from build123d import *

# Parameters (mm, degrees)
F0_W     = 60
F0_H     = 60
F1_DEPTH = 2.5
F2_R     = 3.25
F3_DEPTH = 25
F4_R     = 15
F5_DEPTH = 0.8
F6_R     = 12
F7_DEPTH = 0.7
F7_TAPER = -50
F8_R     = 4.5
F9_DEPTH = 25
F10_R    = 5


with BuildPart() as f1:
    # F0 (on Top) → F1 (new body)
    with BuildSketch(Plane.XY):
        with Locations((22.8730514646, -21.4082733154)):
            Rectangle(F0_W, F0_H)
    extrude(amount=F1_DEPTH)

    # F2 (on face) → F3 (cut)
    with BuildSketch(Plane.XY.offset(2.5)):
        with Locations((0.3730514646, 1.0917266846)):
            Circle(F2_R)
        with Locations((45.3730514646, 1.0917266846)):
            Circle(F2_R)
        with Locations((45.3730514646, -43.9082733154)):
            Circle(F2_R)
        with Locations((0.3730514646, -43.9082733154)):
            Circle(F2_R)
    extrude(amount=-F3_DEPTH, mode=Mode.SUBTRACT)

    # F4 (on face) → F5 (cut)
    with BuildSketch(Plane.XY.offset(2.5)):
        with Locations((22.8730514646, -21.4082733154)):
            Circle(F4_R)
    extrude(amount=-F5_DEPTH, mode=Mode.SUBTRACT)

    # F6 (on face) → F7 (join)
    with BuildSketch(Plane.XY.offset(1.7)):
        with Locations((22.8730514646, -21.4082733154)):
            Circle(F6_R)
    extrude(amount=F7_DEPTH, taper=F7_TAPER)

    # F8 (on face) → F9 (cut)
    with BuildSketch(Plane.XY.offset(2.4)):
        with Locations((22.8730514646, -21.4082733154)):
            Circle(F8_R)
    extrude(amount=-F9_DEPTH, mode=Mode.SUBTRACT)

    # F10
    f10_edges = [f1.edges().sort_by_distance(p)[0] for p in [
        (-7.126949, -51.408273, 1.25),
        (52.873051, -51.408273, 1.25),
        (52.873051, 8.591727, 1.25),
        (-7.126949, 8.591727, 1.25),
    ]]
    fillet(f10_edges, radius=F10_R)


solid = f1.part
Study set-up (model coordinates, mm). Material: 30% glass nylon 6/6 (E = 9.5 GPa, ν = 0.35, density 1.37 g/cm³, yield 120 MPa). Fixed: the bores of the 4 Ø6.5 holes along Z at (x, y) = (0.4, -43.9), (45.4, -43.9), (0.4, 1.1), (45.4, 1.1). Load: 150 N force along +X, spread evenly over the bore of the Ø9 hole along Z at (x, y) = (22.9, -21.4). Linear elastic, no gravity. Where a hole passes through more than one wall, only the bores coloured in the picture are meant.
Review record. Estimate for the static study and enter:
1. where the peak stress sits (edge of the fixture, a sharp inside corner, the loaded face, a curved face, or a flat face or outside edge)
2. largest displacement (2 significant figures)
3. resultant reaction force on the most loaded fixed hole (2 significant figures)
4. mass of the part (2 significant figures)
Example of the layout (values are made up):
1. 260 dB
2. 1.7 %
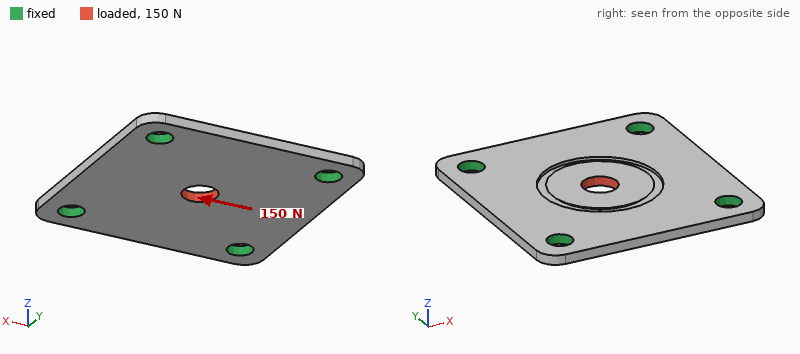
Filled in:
1. the loaded face
2. 5.4 µm
3. 42 N
4. 11 g
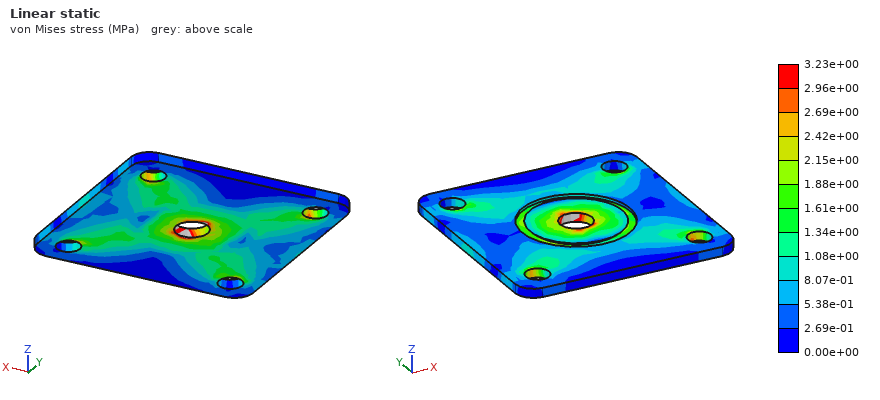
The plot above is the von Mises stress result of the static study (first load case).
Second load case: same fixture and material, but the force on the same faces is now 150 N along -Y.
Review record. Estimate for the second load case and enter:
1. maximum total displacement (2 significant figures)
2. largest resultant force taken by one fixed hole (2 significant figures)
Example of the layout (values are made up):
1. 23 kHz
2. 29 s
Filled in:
1. 5.3 µm
2. 42 N
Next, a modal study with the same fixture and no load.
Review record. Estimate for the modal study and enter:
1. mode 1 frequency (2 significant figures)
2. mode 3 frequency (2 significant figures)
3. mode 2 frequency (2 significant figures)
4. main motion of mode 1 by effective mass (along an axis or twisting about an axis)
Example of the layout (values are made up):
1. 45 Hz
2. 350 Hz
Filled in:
1. 2800 Hz
2. 4300 Hz
3. 4300 Hz
4. along Z
